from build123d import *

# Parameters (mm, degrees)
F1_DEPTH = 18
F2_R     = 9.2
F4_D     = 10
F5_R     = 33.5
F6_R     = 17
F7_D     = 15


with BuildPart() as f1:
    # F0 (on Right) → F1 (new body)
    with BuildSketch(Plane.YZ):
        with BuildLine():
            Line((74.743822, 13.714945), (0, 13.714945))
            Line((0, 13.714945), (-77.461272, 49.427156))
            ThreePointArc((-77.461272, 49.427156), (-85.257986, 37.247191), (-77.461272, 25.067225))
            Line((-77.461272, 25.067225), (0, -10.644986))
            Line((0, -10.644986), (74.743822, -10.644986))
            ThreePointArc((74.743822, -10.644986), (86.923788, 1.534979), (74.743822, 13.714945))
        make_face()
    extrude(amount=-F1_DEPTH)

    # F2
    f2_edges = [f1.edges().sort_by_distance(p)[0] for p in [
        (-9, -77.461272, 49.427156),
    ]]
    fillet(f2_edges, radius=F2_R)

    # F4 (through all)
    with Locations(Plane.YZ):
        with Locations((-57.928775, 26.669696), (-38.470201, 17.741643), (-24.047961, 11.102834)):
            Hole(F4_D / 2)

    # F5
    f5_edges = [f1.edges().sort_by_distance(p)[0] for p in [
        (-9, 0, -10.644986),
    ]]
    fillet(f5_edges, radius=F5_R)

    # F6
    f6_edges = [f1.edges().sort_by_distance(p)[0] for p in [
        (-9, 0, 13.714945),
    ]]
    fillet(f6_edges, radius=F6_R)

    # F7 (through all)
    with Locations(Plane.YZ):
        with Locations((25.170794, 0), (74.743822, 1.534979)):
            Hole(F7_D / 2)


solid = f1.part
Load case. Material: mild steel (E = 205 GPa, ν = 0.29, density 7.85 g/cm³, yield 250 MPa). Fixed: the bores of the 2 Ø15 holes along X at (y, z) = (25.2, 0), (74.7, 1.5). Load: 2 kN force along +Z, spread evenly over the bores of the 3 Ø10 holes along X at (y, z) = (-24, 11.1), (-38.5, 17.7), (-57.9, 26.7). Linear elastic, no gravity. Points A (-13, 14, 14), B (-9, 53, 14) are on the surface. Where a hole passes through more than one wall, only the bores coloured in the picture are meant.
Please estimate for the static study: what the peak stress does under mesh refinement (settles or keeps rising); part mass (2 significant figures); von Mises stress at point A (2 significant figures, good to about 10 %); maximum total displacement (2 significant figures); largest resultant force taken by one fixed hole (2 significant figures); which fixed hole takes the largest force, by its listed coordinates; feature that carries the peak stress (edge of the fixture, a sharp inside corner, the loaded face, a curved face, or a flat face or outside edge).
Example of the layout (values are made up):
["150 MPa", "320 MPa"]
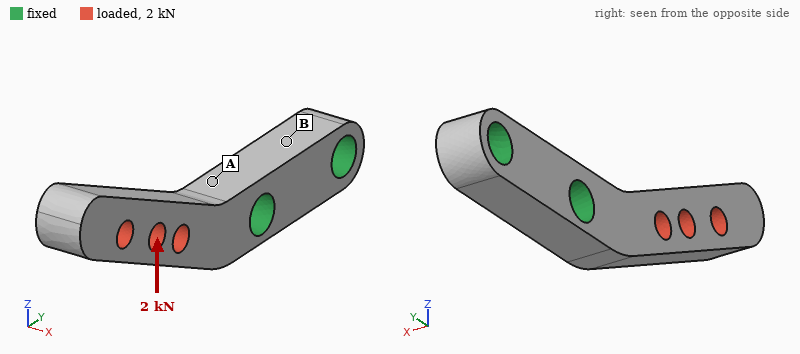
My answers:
["keeps rising", "490 g", "55 MPa", "0.11 mm", "2.2 kN", "(25.2, 0)", "edge of the fixture"]
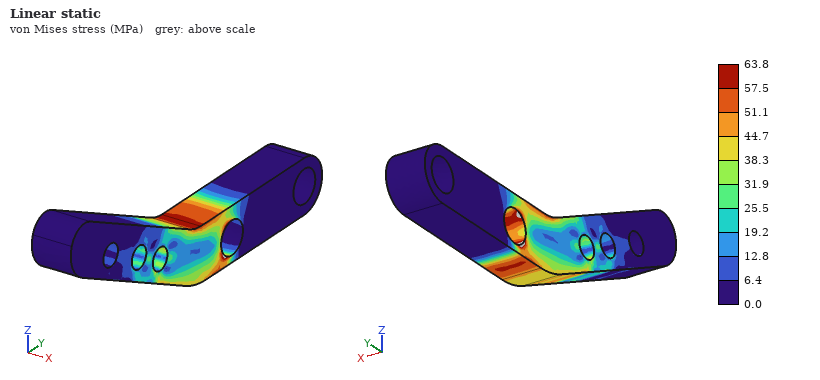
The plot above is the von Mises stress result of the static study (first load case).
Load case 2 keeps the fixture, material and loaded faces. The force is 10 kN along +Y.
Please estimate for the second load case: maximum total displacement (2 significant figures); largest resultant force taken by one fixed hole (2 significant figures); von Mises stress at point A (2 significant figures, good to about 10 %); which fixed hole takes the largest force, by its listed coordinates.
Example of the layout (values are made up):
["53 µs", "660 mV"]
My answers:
["0.19 mm", "9.6 kN", "100 MPa", "(25.2, 0)"]
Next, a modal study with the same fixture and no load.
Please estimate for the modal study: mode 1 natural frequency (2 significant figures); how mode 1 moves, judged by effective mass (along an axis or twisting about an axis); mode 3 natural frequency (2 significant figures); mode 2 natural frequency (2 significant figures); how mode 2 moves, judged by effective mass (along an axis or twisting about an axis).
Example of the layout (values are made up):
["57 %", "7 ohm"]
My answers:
["1200 Hz", "along X", "6000 Hz", "1500 Hz", "along Z"]
